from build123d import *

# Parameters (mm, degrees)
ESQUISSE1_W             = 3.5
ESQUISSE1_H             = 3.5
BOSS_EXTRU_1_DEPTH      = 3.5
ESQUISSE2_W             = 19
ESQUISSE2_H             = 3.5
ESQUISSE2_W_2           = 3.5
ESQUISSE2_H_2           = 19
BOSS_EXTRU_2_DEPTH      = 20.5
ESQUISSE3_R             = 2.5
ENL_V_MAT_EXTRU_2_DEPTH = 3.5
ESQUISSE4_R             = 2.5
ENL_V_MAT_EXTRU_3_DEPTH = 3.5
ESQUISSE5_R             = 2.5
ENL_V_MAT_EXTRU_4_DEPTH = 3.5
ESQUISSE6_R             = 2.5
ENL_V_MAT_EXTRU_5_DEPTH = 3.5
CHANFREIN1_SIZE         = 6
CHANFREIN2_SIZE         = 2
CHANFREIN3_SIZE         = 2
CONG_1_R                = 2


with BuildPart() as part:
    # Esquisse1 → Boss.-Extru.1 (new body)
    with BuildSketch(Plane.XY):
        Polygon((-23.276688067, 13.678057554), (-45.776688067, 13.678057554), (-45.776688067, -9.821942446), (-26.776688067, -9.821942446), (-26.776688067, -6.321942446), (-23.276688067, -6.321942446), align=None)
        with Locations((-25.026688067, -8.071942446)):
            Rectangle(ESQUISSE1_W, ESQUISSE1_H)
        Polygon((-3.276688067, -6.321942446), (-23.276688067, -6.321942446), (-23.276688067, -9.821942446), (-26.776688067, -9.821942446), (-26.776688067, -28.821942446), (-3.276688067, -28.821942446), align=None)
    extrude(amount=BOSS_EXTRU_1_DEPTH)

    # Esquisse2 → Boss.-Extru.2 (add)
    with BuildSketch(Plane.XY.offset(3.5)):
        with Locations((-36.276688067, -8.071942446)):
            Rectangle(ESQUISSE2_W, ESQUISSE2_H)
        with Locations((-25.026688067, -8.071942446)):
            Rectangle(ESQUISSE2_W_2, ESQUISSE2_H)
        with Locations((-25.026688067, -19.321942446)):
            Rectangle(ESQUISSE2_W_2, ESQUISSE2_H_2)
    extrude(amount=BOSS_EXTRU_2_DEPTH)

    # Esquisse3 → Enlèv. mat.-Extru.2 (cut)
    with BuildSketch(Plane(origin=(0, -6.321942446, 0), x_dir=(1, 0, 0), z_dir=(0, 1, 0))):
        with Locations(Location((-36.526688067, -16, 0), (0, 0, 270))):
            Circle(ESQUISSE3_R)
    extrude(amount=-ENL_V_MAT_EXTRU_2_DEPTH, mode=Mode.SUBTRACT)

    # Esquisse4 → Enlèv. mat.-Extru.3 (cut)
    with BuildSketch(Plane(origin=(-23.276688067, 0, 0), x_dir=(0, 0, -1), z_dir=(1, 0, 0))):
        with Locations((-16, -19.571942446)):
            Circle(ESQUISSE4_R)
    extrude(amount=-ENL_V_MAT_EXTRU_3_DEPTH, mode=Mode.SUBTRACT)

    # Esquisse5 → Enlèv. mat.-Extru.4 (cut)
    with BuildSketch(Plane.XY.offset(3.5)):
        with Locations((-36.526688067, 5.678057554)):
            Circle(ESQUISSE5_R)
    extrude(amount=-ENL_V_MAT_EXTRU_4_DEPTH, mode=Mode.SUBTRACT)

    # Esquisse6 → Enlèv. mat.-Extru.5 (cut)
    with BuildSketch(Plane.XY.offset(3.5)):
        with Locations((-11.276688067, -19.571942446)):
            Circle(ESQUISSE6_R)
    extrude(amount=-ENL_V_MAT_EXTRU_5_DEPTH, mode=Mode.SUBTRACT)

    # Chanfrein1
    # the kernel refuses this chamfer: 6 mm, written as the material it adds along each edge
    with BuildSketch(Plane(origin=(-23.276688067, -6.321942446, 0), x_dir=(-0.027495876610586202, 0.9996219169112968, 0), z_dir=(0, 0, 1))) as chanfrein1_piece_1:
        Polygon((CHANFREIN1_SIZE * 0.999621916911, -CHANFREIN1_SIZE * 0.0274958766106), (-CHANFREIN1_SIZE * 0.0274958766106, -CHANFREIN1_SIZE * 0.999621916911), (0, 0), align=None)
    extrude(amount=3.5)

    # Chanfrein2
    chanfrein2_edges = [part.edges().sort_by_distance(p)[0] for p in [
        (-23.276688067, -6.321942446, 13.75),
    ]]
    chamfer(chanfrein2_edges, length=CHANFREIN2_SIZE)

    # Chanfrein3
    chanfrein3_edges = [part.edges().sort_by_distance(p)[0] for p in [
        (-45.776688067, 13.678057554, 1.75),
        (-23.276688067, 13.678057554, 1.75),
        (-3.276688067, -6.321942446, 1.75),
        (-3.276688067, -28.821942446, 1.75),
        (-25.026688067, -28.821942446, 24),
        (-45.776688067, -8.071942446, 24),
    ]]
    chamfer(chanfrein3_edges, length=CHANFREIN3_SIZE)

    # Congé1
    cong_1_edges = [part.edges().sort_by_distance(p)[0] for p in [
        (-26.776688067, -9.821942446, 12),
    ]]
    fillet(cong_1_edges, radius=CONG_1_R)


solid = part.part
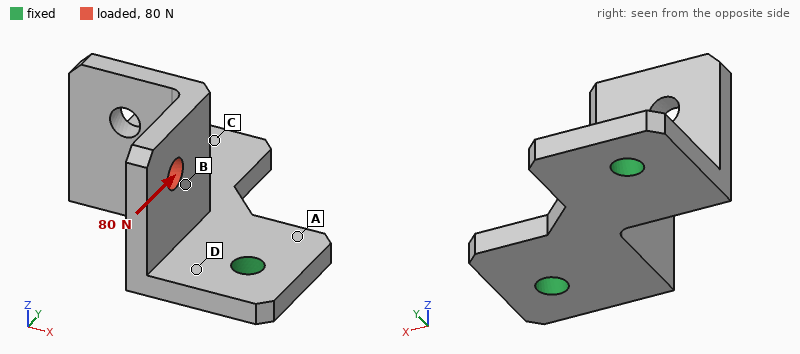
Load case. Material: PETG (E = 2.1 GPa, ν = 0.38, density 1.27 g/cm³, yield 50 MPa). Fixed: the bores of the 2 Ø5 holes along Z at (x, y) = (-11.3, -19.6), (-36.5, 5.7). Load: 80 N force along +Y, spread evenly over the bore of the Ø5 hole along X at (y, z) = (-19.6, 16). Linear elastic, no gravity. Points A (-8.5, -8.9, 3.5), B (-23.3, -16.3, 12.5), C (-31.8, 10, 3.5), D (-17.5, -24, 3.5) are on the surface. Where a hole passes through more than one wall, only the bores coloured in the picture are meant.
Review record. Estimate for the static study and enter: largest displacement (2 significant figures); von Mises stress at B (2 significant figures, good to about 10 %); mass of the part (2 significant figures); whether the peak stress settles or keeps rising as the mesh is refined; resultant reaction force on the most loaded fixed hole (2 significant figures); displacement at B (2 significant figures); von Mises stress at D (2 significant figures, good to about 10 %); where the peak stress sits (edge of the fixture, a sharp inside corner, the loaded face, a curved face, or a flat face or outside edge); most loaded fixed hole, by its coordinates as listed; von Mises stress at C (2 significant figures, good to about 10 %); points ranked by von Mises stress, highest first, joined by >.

0.64 mm
4.2 MPa
8.1 g
keeps rising
54 N
0.28 mm
8.3 MPa
edge of the fixture
(-36.5, 5.7)
2.5 MPa
D > B > C > A
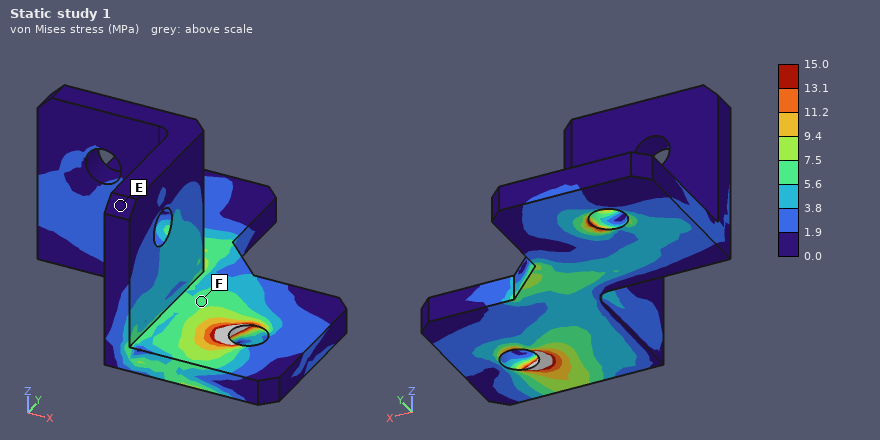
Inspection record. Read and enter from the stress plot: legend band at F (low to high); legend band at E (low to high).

5.6 to 7.5 MPa
0.0 to 1.9 MPa
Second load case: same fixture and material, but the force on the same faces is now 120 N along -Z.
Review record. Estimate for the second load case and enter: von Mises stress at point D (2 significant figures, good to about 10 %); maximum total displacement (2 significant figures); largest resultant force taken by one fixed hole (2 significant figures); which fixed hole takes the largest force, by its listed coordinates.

9.3 MPa
0.64 mm
97 N
(-11.3, -19.6)
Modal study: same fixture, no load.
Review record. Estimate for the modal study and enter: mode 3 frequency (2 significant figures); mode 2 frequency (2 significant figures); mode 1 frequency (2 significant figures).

2100 Hz
2000 Hz
1100 Hz
